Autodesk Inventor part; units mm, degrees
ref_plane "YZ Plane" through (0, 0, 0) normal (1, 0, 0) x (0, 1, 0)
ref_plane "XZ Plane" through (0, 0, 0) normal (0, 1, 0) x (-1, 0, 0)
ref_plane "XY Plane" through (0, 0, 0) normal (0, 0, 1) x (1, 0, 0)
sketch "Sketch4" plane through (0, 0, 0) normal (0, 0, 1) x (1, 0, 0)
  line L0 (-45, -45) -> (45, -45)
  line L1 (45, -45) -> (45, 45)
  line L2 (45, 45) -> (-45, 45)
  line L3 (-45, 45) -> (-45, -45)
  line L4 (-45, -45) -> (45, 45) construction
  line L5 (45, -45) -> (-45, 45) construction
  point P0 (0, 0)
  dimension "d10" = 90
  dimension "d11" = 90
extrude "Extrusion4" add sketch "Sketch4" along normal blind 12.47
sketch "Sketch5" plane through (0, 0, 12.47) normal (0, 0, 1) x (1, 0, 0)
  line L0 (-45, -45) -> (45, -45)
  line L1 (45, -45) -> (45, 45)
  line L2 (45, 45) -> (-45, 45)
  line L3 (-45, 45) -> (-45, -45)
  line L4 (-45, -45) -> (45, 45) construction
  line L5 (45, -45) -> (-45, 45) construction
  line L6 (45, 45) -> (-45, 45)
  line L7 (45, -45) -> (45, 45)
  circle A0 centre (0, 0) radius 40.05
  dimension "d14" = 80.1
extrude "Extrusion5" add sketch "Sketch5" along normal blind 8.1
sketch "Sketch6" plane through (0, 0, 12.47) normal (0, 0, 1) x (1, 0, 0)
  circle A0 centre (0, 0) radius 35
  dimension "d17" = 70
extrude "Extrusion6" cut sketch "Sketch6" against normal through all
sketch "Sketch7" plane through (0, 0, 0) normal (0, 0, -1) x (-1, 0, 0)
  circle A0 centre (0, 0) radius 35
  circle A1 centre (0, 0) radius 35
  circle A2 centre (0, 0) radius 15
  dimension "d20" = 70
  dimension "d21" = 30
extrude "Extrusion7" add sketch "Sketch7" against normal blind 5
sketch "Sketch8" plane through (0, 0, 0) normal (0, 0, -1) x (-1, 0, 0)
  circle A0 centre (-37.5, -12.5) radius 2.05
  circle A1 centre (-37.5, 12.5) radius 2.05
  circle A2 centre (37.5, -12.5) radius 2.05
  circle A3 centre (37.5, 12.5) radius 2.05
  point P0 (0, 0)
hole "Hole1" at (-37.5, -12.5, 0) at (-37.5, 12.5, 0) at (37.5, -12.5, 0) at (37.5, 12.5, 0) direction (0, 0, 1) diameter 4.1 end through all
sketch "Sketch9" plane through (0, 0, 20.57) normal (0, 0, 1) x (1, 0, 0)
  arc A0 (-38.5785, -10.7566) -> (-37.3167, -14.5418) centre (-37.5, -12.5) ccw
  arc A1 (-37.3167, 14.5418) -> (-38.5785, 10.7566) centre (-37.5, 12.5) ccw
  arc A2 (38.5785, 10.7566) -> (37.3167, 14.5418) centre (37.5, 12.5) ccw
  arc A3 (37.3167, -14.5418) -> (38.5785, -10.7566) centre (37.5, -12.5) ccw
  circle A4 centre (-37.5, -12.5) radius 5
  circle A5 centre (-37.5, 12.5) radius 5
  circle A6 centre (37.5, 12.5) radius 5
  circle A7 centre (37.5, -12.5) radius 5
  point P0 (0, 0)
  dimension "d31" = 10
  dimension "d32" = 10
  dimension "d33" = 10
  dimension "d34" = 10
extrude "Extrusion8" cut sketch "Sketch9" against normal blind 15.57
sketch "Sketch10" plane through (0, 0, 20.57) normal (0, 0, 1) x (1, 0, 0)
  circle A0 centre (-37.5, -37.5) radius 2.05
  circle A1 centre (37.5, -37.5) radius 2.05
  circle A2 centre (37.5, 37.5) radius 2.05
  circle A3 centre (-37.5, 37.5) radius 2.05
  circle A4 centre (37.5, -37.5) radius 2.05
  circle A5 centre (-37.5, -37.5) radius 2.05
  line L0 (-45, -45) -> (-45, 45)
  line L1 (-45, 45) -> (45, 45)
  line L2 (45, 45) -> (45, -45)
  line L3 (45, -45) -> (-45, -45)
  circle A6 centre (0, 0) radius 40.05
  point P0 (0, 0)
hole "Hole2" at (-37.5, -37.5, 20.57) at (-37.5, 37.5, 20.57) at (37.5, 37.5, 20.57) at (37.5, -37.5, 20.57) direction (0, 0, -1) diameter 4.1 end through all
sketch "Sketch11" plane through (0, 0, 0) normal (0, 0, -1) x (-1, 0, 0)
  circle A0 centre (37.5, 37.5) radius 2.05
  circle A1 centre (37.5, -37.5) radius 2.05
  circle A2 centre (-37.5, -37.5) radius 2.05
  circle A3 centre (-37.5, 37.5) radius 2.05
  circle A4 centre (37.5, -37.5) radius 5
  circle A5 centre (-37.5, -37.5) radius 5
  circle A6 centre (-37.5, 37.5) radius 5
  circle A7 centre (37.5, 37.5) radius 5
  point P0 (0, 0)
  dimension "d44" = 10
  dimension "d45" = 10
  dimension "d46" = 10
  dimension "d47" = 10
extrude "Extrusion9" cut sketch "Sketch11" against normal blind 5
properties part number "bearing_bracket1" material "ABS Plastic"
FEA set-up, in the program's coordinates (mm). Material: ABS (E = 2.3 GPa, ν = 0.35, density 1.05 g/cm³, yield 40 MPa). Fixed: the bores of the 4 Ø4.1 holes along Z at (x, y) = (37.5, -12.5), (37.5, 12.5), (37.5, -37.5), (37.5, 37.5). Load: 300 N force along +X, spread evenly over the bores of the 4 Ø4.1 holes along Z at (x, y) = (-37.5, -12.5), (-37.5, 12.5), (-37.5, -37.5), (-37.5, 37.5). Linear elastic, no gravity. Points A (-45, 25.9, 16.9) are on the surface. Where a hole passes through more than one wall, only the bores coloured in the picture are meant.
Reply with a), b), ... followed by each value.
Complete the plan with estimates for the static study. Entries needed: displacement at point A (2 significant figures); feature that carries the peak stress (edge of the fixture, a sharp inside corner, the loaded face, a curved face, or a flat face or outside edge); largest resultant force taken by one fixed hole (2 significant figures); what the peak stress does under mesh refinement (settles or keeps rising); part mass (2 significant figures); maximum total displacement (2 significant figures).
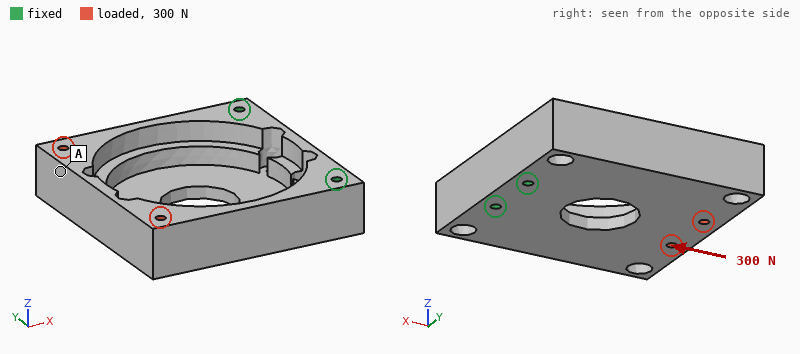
a) 78 µm
b) edge of the fixture
c) 140 N
d) keeps rising
e) 92 g
f) 84 µm
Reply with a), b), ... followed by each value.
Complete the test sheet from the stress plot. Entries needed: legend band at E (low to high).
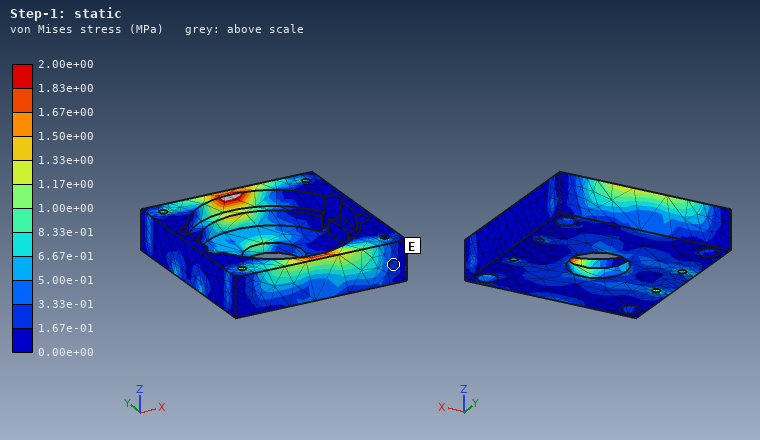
a) 1.67e-01 to 3.33e-01 MPa
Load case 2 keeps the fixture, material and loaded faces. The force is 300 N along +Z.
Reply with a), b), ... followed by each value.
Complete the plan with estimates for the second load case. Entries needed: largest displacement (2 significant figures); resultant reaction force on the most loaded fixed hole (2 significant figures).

a) 1.3 mm
b) 400 N
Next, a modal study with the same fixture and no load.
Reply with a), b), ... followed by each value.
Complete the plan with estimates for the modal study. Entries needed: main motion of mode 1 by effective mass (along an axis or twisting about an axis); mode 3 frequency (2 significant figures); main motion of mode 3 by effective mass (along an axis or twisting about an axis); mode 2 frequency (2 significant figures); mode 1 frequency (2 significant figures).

a) along Z
b) 1400 Hz
c) along Y
d) 670 Hz
e) 450 Hz
